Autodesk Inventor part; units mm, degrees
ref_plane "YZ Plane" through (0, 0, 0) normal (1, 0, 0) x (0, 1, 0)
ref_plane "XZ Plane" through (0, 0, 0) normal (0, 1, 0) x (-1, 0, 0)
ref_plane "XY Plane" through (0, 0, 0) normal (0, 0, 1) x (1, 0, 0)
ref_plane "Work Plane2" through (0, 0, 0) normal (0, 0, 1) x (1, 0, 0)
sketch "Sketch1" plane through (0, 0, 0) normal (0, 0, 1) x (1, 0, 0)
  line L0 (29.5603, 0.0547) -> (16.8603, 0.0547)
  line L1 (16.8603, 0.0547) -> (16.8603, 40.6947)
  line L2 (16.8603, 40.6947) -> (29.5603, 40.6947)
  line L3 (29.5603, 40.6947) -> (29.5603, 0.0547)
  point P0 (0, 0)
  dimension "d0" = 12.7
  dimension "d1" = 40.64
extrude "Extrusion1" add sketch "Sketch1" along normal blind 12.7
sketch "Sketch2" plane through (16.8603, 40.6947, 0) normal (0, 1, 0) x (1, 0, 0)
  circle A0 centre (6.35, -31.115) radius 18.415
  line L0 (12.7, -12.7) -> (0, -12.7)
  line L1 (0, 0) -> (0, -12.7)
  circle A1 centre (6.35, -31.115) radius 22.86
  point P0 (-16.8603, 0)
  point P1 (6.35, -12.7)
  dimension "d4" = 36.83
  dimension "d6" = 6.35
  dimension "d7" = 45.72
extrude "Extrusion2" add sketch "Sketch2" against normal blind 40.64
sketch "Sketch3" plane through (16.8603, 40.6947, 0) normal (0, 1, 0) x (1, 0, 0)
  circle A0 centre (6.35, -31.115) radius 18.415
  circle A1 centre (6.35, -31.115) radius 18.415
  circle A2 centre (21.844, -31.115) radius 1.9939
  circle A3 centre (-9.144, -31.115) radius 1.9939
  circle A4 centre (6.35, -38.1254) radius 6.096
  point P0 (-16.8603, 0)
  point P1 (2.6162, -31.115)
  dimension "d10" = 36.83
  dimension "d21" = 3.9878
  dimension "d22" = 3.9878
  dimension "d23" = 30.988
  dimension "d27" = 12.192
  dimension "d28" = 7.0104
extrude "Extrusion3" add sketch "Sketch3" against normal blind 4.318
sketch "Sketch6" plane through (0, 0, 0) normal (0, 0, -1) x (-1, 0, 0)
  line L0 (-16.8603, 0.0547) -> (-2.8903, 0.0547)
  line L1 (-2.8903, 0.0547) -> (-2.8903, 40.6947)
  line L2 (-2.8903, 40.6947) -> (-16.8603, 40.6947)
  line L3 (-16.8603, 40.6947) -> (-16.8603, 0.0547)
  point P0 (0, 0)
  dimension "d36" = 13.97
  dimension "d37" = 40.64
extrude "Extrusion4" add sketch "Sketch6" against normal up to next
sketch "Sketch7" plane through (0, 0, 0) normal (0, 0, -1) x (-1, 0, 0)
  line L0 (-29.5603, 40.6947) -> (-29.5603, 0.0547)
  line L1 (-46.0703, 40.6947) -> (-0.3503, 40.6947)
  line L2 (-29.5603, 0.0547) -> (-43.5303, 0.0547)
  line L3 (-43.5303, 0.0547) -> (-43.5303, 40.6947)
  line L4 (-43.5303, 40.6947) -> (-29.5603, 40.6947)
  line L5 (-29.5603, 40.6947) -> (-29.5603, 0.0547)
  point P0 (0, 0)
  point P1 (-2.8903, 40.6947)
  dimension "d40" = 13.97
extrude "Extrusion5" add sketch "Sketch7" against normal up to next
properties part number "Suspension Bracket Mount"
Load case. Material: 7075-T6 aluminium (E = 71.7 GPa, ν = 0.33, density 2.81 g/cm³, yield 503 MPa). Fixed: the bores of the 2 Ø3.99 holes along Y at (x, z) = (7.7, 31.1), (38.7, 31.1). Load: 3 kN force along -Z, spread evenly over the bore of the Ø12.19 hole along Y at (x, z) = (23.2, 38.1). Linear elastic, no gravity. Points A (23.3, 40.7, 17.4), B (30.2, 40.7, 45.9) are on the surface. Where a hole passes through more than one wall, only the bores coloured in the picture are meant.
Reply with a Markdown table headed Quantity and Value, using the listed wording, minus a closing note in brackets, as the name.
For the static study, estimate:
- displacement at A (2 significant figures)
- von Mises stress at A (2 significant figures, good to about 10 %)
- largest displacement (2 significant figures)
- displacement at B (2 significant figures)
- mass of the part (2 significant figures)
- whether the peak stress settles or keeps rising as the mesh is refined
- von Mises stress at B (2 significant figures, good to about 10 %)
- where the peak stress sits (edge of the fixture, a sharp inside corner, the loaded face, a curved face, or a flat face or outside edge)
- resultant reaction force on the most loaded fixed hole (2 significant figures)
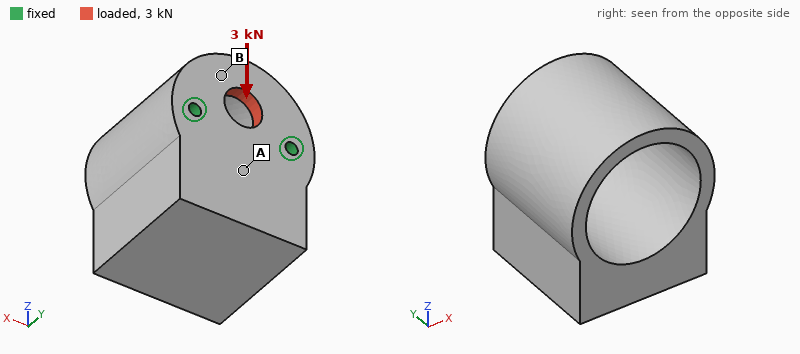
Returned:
| Quantity | Value |
|---|---|
| displacement at A | 2.9 µm |
| von Mises stress at A | 6.5 MPa |
| largest displacement | 8.7 µm |
| displacement at B | 6.0 µm |
| mass of the part | 130 g |
| whether the peak stress settles or keeps rising as the mesh is refined | keeps rising |
| von Mises stress at B | 18 MPa |
| where the peak stress sits | edge of the fixture |
| resultant reaction force on the most loaded fixed hole | 1.5 kN |
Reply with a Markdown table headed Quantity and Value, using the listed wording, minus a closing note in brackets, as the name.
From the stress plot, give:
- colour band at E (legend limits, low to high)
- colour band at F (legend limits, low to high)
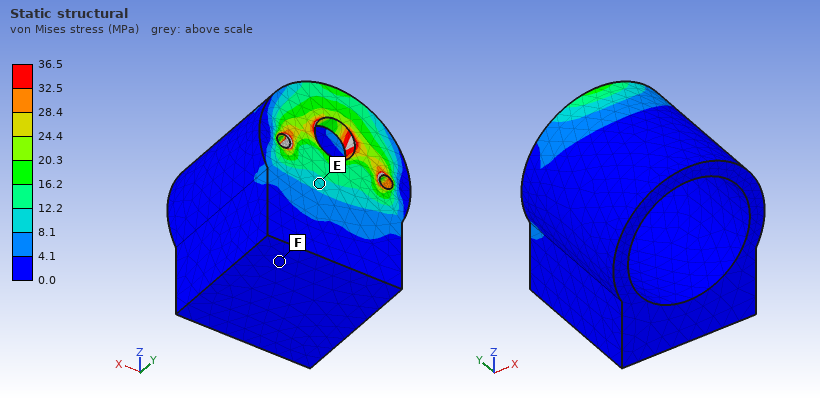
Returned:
| Quantity | Value |
|---|---|
| colour band at E | 8.1 to 12.2 MPa |
| colour band at F | 0.0 to 4.1 MPa |
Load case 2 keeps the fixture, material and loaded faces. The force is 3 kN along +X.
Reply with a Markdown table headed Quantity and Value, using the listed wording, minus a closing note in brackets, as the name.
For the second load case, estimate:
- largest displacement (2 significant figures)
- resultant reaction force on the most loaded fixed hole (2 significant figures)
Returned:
| Quantity | Value |
|---|---|
| largest displacement | 12 µm |
| resultant reaction force on the most loaded fixed hole | 1.6 kN |
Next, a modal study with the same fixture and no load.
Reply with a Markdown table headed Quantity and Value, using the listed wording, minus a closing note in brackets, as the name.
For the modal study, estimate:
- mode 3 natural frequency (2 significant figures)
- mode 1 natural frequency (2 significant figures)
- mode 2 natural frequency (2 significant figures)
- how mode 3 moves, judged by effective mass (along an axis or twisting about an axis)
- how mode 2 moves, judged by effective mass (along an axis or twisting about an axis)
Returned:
| Quantity | Value |
|---|---|
| mode 3 natural frequency | 8100 Hz |
| mode 1 natural frequency | 1400 Hz |
| mode 2 natural frequency | 4600 Hz |
| how mode 3 moves, judged by effective mass | along Y |
| how mode 2 moves, judged by effective mass | along X |
